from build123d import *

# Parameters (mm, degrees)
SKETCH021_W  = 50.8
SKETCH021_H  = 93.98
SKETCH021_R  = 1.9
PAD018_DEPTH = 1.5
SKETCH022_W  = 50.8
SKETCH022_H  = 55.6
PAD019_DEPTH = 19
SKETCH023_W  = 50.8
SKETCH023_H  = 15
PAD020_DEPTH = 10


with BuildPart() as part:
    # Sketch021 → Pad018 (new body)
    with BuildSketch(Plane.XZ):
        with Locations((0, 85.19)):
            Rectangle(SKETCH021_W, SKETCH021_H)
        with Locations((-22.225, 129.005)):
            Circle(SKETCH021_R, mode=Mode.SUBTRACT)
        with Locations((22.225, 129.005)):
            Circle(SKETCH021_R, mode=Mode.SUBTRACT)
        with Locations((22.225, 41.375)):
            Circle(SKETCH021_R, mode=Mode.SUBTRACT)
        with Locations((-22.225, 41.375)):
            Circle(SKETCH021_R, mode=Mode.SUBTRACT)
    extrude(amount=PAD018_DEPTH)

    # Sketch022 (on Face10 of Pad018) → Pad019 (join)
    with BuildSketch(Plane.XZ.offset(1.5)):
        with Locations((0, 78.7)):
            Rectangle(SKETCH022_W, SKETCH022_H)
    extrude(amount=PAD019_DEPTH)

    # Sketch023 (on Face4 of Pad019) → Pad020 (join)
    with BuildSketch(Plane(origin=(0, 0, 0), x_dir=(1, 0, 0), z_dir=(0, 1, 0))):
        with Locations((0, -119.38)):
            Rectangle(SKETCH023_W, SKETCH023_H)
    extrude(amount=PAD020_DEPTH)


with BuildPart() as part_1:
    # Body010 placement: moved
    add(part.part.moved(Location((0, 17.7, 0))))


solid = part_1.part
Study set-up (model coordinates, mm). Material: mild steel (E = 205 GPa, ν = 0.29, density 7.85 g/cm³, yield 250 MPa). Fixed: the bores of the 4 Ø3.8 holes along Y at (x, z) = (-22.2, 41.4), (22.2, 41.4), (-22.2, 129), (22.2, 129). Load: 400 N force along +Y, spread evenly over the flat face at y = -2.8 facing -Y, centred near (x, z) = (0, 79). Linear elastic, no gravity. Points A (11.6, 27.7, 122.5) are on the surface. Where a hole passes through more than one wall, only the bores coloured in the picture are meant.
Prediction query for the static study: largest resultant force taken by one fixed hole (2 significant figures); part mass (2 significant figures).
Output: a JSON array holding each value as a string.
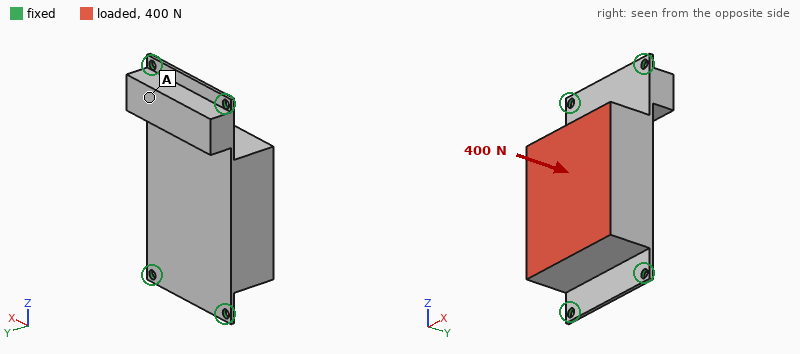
["140 N", "540 g"]
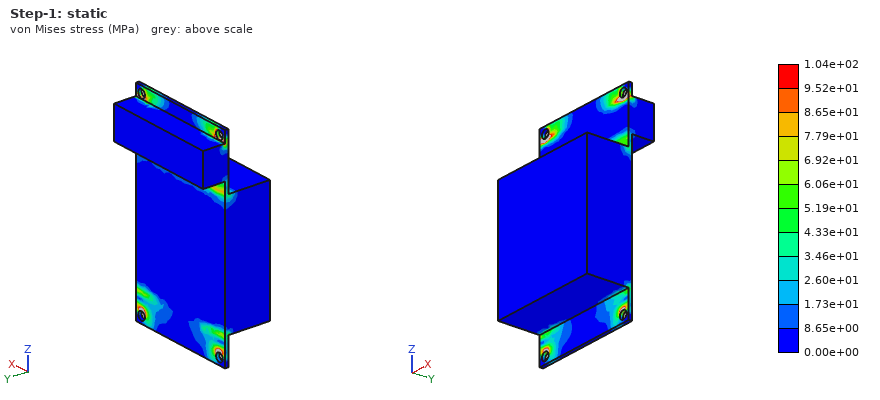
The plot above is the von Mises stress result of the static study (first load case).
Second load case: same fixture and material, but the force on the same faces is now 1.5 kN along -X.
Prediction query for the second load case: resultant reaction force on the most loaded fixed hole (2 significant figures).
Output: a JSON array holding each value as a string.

["690 N"]
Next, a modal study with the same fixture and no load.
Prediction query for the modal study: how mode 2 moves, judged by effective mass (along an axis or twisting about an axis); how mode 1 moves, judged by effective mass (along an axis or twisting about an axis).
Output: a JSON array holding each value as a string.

["along X", "along Y"]
